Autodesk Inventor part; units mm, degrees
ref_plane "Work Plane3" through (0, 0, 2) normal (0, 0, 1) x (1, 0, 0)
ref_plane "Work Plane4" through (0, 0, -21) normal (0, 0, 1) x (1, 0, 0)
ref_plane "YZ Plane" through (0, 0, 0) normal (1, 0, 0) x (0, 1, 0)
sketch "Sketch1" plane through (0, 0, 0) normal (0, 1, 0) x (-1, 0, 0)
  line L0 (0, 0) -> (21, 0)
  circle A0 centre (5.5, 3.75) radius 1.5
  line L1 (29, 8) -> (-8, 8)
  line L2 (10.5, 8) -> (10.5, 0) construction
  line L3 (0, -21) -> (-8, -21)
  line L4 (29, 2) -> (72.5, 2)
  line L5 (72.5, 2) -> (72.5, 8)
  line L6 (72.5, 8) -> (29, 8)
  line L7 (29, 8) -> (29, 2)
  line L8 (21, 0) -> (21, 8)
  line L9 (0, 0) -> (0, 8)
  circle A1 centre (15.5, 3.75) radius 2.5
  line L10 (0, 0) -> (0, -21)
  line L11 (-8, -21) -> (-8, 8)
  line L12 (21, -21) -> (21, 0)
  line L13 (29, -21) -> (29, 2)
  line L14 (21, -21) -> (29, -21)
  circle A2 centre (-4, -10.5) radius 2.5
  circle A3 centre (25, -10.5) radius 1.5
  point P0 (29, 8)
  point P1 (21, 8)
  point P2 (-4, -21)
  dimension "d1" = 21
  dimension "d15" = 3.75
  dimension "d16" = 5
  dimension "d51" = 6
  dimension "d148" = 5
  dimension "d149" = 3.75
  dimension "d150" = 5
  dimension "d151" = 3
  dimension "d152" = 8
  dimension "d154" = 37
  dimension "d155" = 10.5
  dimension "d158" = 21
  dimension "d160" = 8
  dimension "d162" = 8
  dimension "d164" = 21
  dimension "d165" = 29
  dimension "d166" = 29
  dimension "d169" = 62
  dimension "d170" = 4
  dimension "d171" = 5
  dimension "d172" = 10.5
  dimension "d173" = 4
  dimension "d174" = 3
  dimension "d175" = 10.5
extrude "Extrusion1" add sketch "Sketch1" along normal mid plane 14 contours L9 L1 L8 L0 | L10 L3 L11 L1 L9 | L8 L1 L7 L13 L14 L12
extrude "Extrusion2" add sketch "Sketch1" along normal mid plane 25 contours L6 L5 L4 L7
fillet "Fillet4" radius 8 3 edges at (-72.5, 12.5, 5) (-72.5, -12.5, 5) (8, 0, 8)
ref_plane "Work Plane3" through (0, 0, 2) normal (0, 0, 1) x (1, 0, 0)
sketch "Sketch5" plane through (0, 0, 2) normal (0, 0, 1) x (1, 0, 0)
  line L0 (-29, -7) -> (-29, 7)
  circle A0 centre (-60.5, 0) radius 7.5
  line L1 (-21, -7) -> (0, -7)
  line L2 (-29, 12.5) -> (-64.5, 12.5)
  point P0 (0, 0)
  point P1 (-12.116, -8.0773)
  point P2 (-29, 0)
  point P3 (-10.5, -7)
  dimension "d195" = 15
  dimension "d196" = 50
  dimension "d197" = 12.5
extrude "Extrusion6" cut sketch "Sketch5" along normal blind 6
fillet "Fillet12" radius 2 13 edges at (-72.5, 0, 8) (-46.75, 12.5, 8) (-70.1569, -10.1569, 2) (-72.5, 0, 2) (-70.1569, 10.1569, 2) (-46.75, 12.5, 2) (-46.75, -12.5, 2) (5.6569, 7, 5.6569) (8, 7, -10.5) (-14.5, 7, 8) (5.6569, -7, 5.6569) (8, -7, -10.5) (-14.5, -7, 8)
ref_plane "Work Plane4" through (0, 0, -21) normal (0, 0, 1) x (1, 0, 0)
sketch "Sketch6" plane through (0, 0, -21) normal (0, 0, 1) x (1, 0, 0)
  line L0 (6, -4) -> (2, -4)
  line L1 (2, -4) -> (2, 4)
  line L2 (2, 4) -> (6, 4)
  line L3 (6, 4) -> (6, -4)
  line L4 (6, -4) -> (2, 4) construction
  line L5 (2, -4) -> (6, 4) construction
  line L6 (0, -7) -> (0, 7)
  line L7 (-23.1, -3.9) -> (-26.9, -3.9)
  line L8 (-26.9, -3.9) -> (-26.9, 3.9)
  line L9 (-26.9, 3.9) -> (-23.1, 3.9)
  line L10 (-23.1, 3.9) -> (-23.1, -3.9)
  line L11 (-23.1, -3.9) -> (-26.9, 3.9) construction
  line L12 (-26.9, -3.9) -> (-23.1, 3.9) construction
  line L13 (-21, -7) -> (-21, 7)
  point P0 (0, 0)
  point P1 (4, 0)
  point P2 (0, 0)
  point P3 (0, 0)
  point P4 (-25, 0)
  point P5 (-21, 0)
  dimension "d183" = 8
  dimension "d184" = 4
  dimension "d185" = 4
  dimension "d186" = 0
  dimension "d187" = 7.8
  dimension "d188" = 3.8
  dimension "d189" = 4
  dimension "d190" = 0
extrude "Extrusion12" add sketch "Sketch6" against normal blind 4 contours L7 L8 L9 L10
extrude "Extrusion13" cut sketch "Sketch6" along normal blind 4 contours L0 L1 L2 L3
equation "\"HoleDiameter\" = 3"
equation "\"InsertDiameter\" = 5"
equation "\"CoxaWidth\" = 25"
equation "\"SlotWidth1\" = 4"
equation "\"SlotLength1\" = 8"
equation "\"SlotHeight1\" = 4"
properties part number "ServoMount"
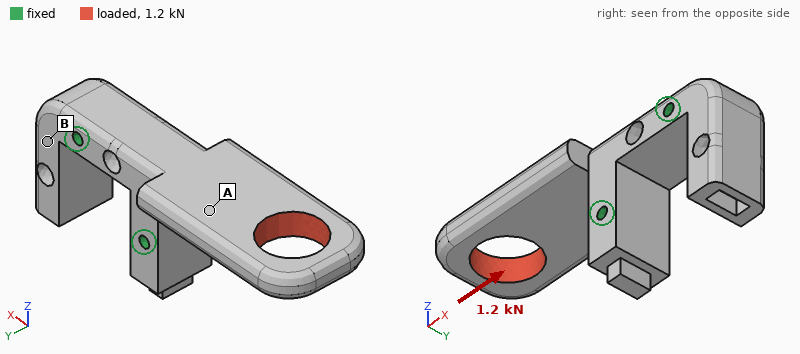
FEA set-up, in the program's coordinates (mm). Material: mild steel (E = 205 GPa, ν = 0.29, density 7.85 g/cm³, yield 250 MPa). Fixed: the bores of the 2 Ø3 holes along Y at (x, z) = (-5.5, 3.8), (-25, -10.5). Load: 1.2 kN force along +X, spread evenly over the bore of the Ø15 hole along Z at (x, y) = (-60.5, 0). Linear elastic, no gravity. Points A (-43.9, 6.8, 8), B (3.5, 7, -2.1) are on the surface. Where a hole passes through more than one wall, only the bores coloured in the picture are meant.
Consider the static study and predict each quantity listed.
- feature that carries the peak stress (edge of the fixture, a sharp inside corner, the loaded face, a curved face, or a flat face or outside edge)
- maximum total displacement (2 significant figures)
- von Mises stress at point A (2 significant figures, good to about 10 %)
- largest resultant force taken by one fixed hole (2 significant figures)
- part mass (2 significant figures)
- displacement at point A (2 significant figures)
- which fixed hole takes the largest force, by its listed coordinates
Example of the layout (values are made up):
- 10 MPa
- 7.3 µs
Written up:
- a curved face
- 9.0 µm
- 9.2 MPa
- 1.1 kN
- 100 g
- 4.2 µm
- (-5.5, 3.8)
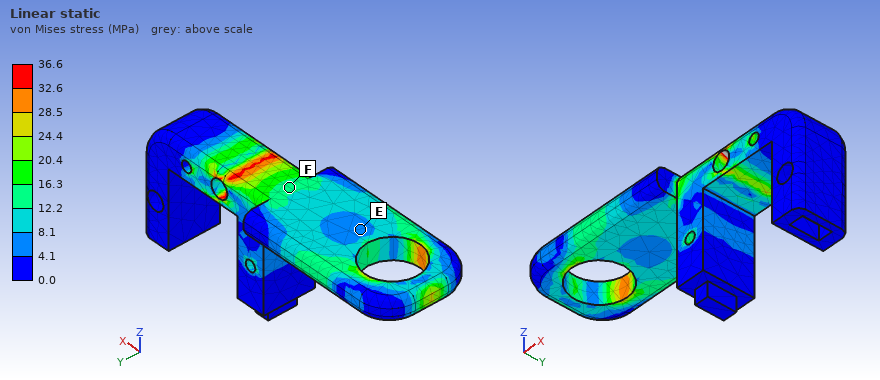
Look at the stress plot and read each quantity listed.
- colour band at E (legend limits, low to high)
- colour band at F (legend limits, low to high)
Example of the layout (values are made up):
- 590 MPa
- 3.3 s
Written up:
- 4.1 to 8.1 MPa
- 12.2 to 16.3 MPa
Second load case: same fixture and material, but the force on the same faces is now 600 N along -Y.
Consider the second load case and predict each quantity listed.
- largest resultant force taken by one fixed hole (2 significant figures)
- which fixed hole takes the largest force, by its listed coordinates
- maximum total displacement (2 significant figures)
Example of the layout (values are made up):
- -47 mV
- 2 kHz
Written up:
- 1.1 kN
- (-25, -10.5)
- 74 µm
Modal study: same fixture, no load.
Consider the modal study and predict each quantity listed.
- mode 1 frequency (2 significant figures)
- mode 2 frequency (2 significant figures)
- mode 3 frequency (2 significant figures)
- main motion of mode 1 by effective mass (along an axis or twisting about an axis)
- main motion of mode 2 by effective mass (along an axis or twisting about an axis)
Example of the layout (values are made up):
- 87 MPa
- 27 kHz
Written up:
- 2300 Hz
- 3500 Hz
- 6800 Hz
- along Z
- along Y
